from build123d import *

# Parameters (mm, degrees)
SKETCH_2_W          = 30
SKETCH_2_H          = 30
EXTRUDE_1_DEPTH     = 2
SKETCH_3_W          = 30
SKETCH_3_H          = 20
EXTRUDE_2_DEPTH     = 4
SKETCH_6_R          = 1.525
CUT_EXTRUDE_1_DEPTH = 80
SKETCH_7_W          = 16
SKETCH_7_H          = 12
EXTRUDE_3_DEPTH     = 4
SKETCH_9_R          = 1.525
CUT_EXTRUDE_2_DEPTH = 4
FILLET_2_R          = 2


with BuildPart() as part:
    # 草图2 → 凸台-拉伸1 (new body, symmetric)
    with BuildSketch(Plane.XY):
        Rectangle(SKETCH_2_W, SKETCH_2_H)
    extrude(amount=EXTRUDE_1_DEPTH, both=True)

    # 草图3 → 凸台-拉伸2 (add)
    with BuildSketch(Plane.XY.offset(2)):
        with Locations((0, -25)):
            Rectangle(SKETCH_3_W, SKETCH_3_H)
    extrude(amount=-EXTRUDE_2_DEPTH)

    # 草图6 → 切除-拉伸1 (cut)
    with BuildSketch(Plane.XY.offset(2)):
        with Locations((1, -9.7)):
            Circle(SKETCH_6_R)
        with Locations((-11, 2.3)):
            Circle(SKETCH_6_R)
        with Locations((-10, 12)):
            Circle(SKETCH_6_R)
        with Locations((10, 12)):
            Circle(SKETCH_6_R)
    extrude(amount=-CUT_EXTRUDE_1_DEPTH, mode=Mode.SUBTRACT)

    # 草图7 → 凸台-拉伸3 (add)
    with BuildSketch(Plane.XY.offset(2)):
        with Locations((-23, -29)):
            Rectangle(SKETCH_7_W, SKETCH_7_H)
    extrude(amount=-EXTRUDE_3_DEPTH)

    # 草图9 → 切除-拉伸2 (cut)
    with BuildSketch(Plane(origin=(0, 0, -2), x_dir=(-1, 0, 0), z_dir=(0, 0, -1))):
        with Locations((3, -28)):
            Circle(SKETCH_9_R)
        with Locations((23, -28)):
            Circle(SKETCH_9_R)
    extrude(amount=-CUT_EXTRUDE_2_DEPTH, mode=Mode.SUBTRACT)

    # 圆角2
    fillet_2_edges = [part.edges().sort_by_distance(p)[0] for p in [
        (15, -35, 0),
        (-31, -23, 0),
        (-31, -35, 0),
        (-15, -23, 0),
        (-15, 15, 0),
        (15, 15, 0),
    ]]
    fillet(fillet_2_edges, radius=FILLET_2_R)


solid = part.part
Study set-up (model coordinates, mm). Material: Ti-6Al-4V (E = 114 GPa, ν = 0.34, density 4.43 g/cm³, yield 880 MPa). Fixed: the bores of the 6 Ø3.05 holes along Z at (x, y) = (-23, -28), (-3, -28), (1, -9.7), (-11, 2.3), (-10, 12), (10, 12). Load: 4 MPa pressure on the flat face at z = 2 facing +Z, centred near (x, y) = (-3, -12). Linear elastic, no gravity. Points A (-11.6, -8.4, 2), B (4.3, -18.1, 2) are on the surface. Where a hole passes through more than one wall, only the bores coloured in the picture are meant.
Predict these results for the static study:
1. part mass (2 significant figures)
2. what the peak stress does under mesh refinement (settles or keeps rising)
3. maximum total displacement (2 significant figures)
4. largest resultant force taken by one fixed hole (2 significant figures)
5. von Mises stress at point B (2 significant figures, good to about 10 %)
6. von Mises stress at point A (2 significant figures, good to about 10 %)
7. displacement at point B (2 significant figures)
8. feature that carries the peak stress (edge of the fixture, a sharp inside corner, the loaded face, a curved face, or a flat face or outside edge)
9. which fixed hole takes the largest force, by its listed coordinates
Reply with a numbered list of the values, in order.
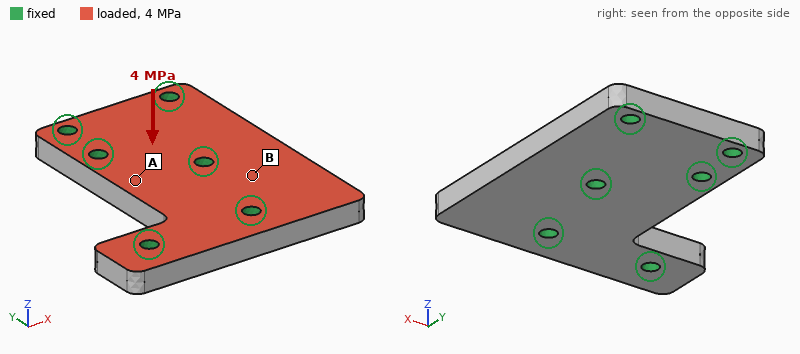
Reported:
1. 29 g
2. keeps rising
3. 70 µm
4. 2.0 kN
5. 71 MPa
6. 20 MPa
7. 15 µm
8. edge of the fixture
9. (1, -9.7)
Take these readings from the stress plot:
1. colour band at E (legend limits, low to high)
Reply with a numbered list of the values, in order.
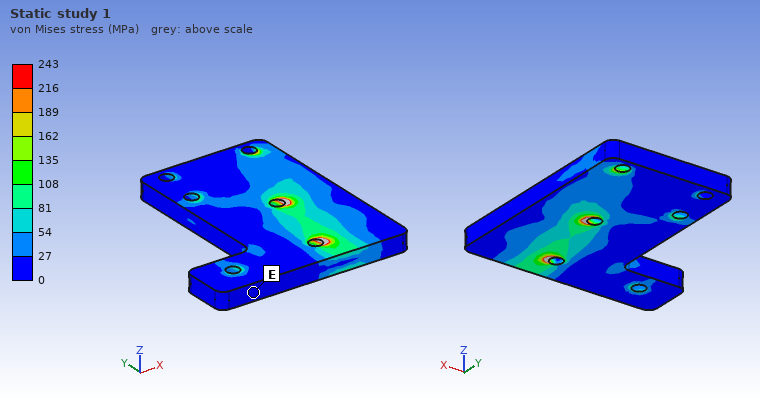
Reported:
1. 0 to 27 MPa
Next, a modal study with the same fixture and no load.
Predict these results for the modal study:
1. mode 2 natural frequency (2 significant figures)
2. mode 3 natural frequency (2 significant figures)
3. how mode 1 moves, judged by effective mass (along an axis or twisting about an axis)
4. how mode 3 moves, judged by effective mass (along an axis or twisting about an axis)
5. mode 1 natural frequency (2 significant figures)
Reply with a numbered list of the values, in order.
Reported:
1. 21 kHz
2. 26 kHz
3. along Z
4. along Z
5. 12 kHz
